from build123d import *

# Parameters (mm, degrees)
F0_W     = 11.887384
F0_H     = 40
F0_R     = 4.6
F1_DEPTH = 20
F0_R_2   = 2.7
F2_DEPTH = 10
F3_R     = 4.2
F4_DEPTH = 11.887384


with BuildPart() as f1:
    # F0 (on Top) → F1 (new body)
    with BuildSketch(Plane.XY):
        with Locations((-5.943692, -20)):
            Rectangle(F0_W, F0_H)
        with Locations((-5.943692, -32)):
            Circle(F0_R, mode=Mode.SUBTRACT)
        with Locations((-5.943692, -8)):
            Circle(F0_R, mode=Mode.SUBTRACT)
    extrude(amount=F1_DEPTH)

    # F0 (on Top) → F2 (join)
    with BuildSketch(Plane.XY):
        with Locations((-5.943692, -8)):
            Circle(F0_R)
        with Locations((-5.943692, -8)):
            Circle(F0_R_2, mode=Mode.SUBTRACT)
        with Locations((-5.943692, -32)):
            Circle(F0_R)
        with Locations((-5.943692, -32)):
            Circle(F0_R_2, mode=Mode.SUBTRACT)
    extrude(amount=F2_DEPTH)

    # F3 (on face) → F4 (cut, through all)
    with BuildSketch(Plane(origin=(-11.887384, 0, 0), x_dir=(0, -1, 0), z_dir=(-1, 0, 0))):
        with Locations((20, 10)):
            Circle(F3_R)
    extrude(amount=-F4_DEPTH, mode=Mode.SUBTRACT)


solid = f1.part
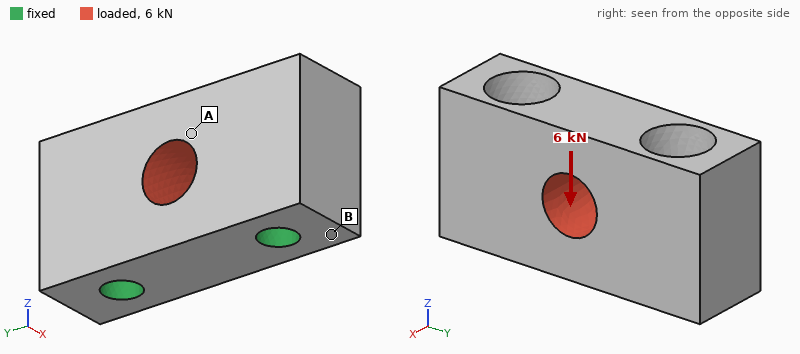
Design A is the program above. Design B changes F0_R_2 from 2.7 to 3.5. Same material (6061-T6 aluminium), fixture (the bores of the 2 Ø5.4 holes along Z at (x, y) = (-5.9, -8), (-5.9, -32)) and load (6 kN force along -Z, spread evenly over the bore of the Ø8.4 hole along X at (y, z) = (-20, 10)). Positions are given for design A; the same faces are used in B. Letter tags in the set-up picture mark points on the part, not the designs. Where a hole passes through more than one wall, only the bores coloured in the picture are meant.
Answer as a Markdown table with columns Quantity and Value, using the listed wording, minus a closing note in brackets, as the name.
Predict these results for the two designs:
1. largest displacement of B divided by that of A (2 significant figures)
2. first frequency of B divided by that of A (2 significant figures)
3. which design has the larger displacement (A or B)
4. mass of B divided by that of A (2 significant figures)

| Quantity | Value |
|---|---|
| largest displacement of B divided by that of A | 0.88 |
| first frequency of B divided by that of A | 1.1 |
| which design has the larger displacement | A |
| mass of B divided by that of A | 0.96 |
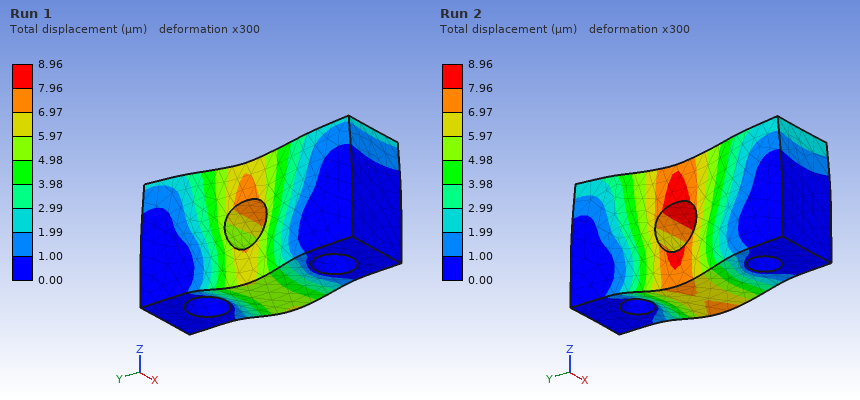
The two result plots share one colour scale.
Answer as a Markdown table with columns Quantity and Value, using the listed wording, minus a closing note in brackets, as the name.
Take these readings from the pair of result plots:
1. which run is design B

| Quantity | Value |
|---|---|
| which run is design B | Run 1 |
